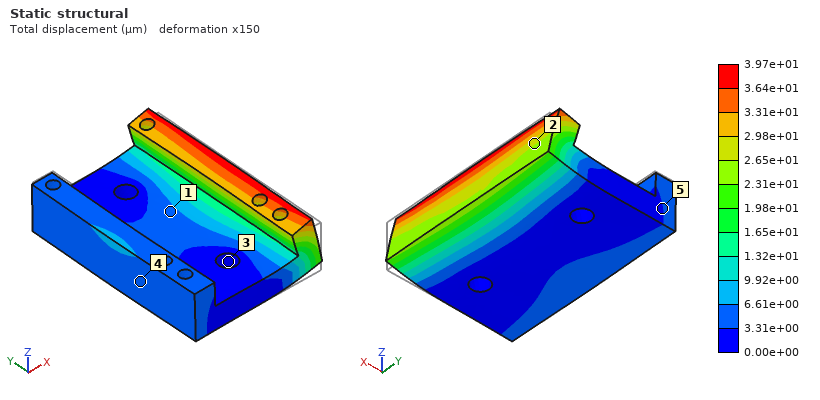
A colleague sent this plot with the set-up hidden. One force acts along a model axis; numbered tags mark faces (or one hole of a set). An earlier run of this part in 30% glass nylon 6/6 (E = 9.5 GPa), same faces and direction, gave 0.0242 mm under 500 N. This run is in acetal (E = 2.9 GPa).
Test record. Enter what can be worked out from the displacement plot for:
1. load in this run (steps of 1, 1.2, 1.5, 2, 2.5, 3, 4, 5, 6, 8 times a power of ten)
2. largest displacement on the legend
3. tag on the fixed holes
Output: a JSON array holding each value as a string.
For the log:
["250 N", "3.97e+01 µm", "3"]
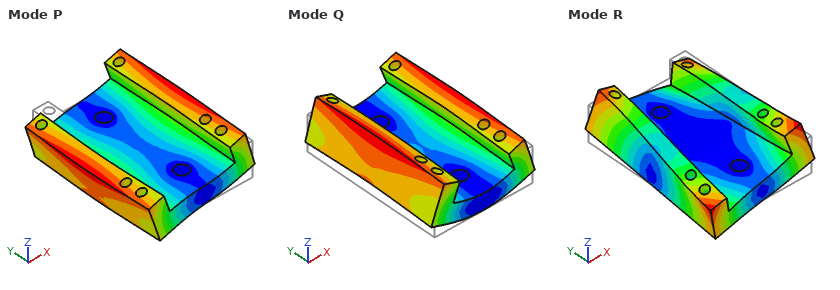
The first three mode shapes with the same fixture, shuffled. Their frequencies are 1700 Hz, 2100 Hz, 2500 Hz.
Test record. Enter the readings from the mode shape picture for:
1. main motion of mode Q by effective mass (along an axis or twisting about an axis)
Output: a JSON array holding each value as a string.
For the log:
["along Z"]
